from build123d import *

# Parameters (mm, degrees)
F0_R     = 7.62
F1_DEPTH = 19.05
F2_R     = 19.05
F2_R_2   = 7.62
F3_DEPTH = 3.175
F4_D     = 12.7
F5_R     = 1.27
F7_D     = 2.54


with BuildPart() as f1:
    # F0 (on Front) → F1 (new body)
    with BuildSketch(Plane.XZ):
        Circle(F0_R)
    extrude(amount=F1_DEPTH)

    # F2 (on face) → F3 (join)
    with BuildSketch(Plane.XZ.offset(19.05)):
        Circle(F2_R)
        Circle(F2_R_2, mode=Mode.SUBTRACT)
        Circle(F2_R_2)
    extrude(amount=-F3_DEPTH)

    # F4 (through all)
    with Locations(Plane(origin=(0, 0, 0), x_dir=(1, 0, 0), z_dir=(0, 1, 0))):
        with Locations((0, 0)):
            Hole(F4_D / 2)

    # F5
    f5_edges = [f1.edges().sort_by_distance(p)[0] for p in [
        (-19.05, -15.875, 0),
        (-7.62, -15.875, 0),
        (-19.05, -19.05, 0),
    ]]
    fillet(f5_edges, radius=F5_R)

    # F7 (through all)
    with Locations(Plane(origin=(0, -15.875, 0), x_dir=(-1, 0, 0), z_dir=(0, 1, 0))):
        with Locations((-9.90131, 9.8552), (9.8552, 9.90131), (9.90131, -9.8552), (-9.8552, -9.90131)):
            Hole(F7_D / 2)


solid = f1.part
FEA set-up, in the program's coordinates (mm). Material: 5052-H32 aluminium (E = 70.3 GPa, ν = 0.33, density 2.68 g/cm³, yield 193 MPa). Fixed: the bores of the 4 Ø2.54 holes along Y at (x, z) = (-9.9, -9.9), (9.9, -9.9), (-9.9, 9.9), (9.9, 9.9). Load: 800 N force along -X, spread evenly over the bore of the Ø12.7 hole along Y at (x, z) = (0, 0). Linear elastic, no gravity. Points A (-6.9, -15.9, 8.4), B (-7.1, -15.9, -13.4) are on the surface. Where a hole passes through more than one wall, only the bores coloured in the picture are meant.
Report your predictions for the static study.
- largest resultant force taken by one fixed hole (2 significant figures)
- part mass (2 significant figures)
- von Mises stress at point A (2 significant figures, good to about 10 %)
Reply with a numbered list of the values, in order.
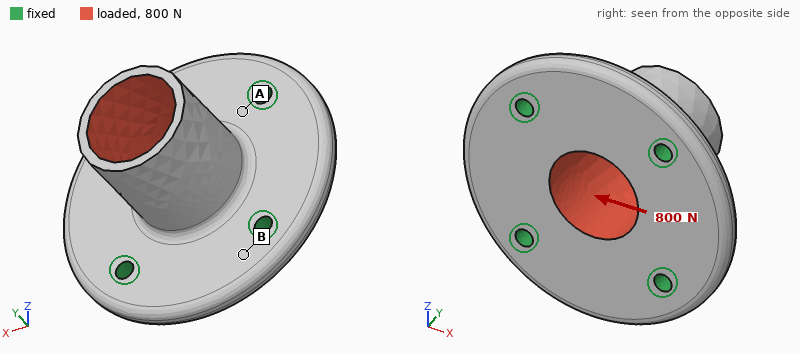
1. 280 N
2. 11 g
3. 17 MPa
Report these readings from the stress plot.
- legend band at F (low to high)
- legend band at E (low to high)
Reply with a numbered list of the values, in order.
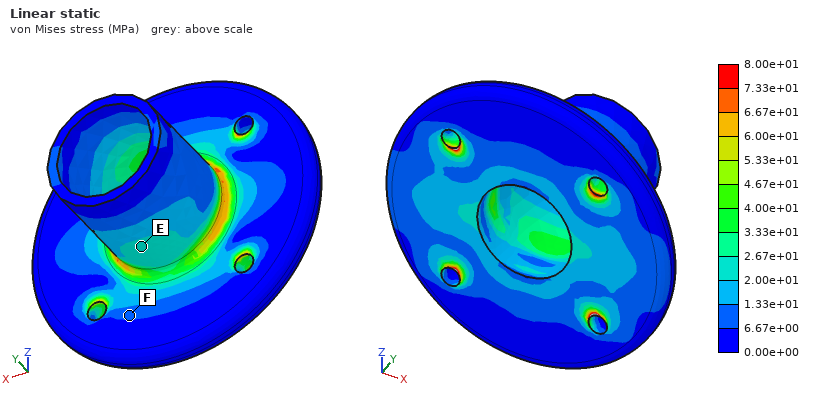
1. 6.67e+00 to 1.33e+01 MPa
2. 2.00e+01 to 2.67e+01 MPa
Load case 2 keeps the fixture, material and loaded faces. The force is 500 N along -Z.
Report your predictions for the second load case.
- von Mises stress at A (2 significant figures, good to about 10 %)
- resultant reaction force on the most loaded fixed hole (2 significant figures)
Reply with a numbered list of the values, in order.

1. 5.7 MPa
2. 170 N
